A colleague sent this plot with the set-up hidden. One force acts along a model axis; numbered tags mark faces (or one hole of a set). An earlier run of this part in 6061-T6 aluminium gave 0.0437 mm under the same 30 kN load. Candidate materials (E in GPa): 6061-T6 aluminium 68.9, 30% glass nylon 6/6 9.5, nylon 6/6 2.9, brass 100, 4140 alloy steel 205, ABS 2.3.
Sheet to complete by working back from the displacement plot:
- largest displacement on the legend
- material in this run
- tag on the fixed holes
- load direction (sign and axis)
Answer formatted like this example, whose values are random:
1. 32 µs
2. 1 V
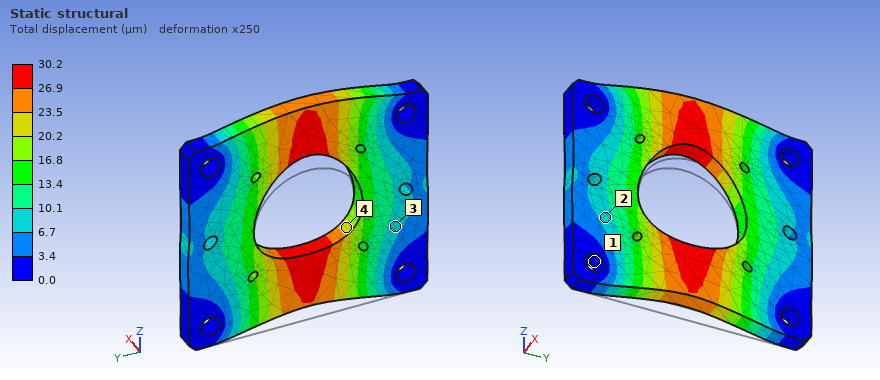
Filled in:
1. 30.2 µm
2. brass
3. 1
4. +Z
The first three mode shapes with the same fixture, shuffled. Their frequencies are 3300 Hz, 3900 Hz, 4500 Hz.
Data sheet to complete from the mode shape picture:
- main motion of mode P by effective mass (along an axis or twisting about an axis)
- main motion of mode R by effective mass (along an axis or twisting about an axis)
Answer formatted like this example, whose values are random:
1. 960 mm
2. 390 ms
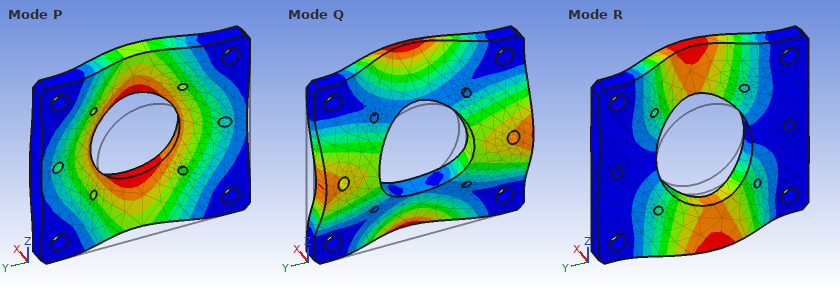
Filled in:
1. along X
2. twisting about Y
